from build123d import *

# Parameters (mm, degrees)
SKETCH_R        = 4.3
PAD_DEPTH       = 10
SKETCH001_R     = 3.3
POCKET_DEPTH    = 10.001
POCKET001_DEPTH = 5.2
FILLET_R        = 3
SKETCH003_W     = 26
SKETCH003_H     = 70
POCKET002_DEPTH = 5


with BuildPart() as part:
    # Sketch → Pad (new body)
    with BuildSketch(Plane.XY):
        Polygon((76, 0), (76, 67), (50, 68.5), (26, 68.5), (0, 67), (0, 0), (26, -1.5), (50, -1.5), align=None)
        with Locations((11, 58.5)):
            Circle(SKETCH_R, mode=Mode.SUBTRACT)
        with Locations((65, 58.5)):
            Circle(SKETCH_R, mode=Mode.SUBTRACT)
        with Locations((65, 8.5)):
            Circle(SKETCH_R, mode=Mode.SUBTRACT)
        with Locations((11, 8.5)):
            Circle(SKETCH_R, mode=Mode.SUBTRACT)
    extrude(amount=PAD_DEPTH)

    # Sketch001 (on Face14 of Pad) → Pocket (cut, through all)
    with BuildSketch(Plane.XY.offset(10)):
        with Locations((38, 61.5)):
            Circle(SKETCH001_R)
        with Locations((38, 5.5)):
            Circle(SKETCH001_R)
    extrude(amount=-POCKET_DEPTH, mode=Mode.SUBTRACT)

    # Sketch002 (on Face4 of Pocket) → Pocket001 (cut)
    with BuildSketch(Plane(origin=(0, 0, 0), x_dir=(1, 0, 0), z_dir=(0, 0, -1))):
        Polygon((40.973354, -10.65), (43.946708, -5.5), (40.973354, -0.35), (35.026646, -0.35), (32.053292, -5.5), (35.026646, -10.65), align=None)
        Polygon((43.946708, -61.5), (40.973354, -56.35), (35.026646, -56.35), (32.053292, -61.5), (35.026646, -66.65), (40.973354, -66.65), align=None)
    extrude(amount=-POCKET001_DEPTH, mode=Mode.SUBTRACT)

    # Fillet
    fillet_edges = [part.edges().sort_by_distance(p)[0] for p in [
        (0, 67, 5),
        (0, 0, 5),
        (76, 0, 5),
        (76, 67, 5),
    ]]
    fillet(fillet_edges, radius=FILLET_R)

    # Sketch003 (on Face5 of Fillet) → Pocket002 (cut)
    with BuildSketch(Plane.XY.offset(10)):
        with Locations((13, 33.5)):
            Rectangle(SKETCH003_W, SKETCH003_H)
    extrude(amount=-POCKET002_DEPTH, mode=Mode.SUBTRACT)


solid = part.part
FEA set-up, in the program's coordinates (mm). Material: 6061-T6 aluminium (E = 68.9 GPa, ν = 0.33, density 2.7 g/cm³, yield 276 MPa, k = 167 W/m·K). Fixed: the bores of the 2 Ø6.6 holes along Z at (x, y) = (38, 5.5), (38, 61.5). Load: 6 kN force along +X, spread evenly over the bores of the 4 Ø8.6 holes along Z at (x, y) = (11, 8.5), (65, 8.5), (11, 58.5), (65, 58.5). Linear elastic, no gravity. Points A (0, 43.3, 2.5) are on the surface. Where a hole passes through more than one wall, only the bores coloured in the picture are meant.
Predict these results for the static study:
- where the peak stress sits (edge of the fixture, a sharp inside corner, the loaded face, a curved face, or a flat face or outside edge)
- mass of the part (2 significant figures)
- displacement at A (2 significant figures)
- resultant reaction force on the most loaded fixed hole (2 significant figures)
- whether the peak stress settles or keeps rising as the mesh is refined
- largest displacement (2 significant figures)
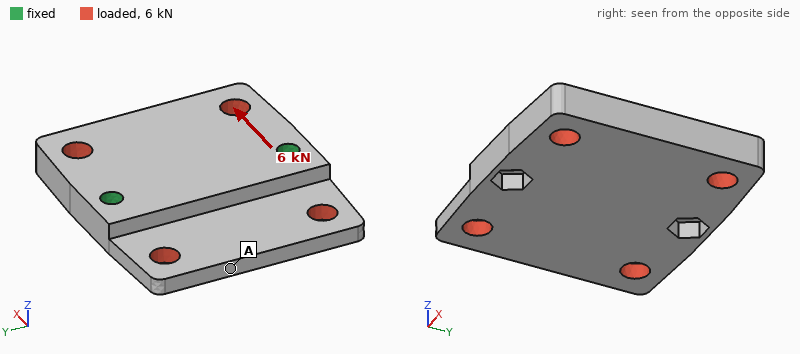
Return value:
edge of the fixture
110 g
51 µm
3.0 kN
keeps rising
53 µm
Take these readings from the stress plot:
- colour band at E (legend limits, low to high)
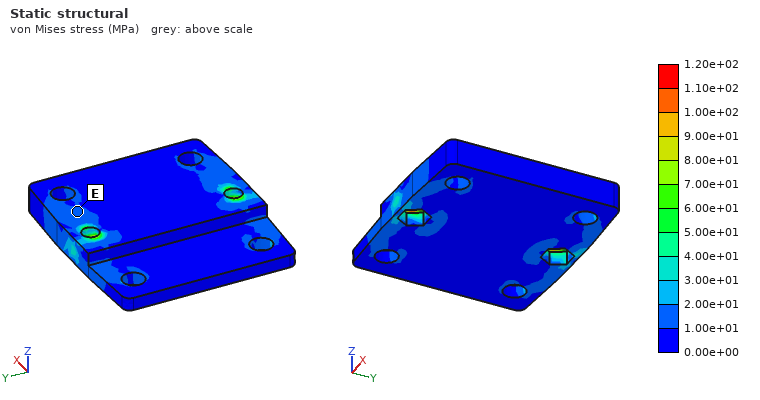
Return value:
1.00e+01 to 2.00e+01 MPa
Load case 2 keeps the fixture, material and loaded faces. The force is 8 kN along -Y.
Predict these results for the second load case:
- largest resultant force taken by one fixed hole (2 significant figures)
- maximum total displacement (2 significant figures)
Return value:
4.2 kN
21 µm
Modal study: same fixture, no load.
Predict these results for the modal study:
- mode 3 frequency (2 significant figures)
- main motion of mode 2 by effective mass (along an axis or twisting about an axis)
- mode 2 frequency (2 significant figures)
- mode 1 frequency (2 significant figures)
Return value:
6100 Hz
along Z
4500 Hz
2700 Hz
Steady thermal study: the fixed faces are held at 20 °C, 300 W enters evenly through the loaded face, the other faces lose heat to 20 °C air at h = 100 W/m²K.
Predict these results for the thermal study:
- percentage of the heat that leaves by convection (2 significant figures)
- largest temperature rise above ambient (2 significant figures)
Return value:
19 %
80 K
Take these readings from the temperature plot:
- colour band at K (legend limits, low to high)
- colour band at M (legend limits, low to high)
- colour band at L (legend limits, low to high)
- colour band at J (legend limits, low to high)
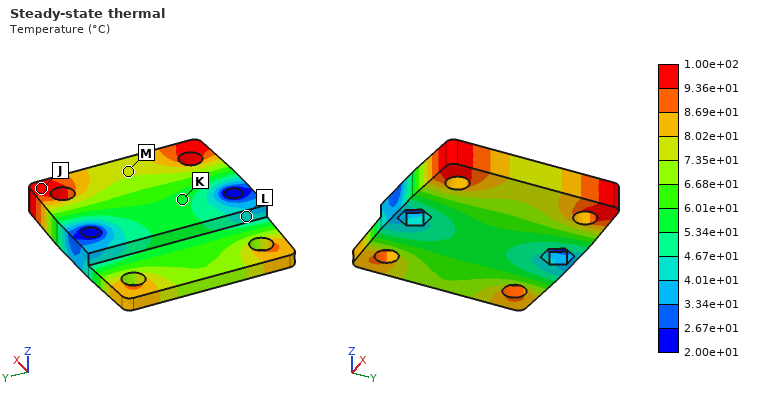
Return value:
5.34e+01 to 6.01e+01 °C
7.35e+01 to 8.02e+01 °C
4.01e+01 to 4.67e+01 °C
9.36e+01 to 1.00e+02 °C
